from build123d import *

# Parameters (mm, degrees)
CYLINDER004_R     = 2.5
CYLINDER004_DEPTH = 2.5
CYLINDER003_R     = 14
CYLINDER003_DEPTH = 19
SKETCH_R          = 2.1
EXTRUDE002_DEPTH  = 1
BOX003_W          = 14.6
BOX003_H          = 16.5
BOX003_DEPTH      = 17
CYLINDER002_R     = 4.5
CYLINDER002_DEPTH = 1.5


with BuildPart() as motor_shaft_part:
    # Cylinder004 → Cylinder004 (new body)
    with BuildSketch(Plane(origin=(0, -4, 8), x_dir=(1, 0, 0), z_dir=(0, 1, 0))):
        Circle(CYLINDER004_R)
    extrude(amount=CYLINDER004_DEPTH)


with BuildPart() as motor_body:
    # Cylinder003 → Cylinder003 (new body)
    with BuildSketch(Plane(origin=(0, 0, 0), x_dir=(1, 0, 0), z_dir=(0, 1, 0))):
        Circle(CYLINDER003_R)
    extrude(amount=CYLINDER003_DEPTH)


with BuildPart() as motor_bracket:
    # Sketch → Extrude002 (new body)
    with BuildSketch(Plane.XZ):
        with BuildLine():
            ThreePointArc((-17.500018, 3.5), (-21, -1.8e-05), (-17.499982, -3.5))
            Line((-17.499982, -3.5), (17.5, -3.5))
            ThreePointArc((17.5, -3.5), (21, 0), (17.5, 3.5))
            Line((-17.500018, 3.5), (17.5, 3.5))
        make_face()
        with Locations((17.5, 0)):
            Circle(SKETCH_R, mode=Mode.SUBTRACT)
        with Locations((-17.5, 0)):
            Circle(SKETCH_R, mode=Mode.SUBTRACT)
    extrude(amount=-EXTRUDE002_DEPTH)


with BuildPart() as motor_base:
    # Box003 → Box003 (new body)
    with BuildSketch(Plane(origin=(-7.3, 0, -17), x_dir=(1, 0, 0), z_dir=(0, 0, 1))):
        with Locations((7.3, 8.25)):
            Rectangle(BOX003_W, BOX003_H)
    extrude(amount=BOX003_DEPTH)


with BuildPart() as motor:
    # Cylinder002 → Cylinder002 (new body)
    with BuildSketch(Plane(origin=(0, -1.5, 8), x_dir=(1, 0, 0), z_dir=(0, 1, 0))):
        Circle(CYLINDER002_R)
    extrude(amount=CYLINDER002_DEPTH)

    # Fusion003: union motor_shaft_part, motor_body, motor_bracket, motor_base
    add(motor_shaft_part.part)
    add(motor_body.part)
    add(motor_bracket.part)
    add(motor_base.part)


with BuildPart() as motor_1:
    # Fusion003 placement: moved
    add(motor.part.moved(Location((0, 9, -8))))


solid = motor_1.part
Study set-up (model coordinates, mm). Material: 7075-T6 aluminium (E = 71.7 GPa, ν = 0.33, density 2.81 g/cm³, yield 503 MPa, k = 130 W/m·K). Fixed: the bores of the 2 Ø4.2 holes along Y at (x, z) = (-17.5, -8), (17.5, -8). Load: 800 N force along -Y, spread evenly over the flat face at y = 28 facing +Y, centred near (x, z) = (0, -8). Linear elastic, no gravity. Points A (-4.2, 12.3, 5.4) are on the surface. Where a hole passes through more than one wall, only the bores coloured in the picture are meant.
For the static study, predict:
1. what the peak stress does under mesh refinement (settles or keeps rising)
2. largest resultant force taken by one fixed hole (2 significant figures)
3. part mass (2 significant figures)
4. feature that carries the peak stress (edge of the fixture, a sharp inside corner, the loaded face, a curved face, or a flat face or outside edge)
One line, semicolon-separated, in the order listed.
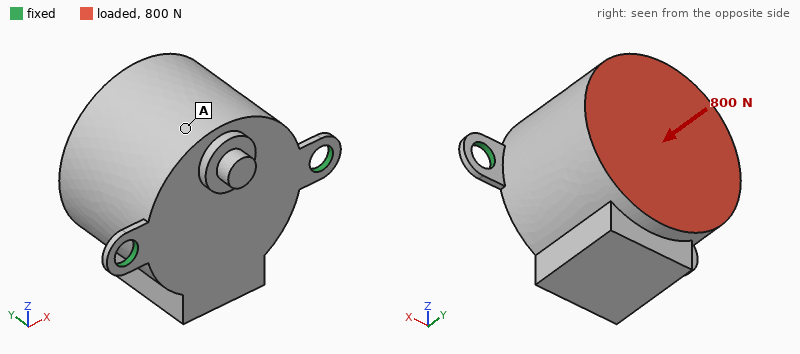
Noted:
keeps rising; 460 N; 36 g; edge of the fixture
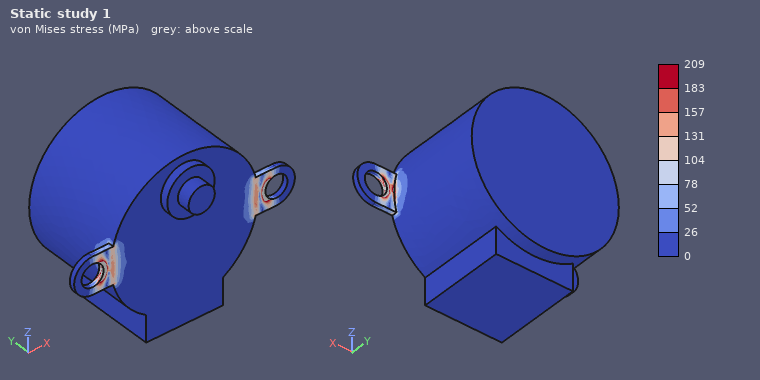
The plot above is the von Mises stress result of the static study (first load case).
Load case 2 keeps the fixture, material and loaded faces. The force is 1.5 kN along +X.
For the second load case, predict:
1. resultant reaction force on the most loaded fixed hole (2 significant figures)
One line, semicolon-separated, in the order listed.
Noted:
1.2 kN
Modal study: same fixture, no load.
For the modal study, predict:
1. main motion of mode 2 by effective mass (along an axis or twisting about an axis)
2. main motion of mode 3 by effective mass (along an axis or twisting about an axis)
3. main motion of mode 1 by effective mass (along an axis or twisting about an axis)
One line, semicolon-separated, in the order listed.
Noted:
along Y; along X; along Z
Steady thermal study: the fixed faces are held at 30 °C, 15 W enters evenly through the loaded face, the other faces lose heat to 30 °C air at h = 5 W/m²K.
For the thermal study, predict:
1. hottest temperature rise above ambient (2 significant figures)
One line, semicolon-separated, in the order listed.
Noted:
31 K
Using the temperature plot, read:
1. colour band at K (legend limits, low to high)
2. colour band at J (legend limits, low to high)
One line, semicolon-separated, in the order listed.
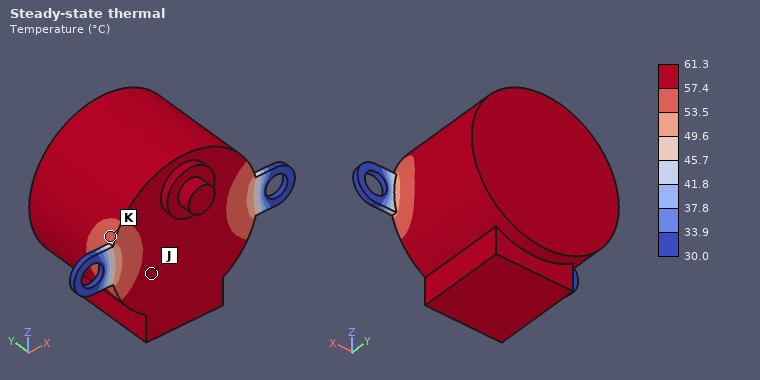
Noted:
53.5 to 57.4 °C; 57.4 to 61.3 °C
